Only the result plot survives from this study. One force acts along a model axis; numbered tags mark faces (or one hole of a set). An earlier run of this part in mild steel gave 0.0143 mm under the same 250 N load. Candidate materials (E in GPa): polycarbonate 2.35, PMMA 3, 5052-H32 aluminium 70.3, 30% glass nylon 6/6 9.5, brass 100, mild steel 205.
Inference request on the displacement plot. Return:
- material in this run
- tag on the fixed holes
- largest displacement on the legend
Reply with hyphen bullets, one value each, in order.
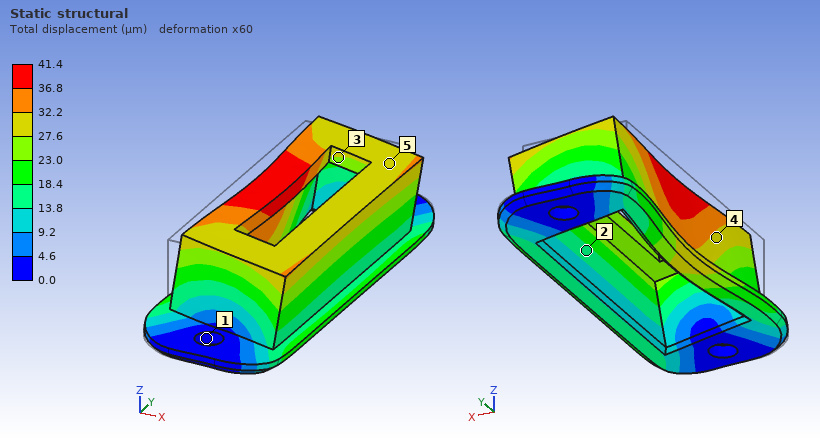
- 5052-H32 aluminium
- 1
- 41.4 µm
